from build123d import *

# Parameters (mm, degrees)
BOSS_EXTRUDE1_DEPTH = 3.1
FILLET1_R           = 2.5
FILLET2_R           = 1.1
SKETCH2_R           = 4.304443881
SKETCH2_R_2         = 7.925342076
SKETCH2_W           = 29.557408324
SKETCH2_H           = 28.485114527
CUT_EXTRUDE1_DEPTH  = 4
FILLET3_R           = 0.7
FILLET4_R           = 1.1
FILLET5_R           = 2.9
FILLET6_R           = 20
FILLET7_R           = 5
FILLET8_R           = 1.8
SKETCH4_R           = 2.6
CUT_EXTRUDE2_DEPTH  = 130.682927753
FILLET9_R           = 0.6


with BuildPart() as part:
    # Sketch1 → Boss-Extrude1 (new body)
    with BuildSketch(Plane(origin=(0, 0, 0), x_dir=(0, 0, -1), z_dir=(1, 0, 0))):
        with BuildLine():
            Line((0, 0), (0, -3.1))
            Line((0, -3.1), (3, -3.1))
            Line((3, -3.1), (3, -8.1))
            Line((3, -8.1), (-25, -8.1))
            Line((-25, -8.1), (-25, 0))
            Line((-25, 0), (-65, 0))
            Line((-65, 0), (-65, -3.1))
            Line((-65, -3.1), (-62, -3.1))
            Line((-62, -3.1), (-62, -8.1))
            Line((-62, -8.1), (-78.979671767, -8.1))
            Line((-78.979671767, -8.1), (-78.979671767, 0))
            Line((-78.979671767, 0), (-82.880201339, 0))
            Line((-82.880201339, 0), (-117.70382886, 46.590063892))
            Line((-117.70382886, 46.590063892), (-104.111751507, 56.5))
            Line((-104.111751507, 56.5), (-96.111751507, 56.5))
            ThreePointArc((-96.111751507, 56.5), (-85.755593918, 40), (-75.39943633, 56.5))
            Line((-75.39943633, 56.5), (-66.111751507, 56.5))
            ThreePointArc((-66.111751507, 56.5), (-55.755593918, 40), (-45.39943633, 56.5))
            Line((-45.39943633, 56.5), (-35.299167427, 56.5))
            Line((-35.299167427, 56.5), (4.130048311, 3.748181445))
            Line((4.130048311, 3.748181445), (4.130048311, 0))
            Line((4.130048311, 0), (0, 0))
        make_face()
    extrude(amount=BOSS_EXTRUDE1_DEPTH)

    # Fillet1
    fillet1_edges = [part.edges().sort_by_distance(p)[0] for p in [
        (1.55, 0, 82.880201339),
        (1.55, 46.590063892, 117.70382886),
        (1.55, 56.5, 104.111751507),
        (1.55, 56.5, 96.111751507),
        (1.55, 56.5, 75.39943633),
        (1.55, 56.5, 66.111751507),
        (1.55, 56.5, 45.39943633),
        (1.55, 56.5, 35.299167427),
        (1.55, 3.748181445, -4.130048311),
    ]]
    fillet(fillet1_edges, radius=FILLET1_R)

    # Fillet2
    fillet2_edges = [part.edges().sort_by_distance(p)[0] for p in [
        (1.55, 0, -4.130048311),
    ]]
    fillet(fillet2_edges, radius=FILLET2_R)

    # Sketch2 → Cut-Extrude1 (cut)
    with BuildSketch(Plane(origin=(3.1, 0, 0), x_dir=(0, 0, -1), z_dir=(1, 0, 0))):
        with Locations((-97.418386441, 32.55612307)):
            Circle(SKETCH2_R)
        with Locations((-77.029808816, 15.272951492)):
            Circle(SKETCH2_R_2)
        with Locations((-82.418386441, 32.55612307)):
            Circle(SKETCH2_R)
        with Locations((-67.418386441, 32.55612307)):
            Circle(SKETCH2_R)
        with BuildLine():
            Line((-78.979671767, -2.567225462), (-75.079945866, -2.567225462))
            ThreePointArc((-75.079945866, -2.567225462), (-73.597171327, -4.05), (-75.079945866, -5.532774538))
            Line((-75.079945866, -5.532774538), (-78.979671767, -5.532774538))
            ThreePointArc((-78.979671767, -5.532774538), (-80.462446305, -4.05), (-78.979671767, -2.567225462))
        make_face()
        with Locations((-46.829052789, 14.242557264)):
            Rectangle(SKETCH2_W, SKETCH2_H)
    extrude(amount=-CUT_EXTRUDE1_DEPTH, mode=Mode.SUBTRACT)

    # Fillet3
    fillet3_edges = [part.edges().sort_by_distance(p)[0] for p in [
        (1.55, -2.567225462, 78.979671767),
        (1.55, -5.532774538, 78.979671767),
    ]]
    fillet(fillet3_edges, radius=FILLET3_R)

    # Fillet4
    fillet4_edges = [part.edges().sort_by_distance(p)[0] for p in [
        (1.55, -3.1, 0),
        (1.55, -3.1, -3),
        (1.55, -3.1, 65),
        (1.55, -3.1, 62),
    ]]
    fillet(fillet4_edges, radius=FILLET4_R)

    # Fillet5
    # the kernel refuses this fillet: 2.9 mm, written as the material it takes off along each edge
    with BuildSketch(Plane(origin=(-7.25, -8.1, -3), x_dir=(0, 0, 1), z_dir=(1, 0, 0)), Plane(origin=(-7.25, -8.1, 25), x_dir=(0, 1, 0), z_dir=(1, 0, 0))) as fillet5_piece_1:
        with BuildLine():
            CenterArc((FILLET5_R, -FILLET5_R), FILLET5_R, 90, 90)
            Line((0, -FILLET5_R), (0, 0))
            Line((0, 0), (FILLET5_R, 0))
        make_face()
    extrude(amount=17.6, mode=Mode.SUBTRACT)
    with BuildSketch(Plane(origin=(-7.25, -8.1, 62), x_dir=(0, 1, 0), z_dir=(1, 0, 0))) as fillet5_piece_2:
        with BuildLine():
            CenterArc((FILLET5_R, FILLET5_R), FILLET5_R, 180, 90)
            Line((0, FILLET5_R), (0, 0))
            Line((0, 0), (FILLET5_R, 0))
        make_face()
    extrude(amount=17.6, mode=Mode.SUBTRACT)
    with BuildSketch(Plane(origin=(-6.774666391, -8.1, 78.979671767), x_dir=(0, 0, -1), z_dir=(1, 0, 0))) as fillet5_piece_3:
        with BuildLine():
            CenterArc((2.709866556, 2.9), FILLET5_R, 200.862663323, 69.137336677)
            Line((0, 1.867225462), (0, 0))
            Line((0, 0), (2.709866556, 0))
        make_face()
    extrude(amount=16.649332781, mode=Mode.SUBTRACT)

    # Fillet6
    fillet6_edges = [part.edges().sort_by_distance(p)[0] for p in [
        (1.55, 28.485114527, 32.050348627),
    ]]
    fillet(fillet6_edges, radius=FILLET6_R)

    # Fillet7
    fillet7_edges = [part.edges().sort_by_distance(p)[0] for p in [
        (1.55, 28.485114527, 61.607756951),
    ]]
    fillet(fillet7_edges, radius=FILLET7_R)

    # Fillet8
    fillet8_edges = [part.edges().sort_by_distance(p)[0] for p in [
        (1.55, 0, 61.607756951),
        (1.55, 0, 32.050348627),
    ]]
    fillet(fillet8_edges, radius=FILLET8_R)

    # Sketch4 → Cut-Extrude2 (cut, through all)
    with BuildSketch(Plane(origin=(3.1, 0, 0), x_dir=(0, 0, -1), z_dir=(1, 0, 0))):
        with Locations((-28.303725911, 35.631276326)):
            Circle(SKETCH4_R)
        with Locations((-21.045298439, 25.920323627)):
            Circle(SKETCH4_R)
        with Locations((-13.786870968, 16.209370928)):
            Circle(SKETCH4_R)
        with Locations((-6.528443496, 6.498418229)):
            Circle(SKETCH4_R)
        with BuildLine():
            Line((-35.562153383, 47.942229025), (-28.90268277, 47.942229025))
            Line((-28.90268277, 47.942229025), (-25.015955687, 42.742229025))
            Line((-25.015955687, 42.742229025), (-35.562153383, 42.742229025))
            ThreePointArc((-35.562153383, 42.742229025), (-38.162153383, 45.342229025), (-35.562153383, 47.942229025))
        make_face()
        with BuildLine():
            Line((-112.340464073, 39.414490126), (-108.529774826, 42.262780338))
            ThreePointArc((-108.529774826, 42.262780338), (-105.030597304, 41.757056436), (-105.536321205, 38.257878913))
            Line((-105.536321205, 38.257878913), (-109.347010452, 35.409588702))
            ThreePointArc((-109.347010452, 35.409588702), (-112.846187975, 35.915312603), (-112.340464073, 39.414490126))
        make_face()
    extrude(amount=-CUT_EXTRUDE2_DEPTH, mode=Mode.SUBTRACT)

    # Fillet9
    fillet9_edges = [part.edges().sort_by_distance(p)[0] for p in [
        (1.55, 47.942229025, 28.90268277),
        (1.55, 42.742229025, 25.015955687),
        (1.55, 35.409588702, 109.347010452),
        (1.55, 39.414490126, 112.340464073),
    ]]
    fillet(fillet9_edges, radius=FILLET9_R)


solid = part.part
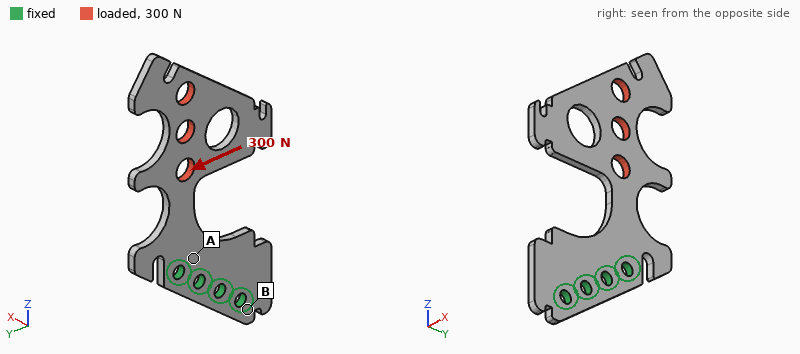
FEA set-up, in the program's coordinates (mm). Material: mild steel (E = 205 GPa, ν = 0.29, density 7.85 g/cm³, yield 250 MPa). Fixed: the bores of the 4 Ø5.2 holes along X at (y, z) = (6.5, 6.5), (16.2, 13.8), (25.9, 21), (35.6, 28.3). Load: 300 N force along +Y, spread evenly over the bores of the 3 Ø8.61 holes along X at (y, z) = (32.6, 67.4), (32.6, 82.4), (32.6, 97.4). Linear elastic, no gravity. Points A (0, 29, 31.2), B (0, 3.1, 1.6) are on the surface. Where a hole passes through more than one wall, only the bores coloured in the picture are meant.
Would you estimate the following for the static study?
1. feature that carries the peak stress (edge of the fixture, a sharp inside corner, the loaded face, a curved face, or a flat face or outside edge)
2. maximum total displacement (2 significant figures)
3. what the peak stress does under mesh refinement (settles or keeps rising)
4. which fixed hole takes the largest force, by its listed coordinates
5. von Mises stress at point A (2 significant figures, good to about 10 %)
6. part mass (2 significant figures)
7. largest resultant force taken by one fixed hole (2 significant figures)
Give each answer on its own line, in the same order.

a sharp inside corner
0.17 mm
keeps rising
(35.6, 28.3)
25 MPa
81 g
920 N
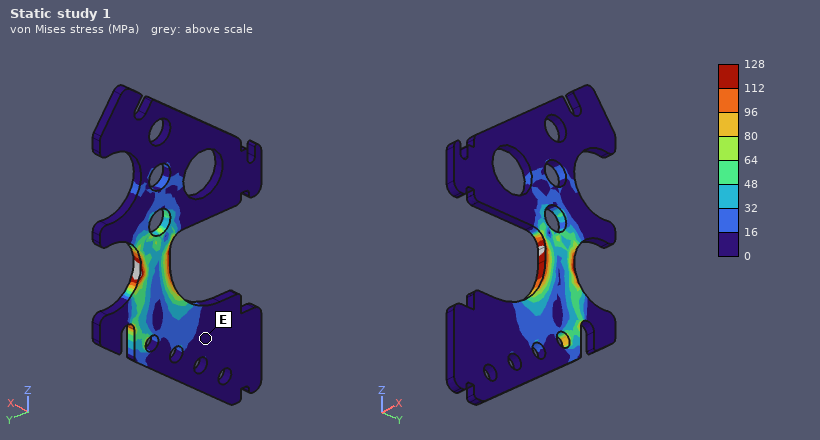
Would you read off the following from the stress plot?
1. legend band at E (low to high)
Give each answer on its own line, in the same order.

0 to 16 MPa
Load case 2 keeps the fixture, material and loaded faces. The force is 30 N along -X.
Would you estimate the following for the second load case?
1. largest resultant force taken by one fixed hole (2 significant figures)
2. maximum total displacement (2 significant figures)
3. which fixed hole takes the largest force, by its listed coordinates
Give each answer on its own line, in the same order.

63 N
0.36 mm
(35.6, 28.3)
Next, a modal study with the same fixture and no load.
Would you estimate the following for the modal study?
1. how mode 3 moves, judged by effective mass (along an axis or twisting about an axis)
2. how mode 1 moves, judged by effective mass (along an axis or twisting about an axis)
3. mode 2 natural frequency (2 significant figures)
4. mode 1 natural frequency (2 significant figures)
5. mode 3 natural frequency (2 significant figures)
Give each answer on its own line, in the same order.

along Y
along X
660 Hz
300 Hz
1200 Hz
